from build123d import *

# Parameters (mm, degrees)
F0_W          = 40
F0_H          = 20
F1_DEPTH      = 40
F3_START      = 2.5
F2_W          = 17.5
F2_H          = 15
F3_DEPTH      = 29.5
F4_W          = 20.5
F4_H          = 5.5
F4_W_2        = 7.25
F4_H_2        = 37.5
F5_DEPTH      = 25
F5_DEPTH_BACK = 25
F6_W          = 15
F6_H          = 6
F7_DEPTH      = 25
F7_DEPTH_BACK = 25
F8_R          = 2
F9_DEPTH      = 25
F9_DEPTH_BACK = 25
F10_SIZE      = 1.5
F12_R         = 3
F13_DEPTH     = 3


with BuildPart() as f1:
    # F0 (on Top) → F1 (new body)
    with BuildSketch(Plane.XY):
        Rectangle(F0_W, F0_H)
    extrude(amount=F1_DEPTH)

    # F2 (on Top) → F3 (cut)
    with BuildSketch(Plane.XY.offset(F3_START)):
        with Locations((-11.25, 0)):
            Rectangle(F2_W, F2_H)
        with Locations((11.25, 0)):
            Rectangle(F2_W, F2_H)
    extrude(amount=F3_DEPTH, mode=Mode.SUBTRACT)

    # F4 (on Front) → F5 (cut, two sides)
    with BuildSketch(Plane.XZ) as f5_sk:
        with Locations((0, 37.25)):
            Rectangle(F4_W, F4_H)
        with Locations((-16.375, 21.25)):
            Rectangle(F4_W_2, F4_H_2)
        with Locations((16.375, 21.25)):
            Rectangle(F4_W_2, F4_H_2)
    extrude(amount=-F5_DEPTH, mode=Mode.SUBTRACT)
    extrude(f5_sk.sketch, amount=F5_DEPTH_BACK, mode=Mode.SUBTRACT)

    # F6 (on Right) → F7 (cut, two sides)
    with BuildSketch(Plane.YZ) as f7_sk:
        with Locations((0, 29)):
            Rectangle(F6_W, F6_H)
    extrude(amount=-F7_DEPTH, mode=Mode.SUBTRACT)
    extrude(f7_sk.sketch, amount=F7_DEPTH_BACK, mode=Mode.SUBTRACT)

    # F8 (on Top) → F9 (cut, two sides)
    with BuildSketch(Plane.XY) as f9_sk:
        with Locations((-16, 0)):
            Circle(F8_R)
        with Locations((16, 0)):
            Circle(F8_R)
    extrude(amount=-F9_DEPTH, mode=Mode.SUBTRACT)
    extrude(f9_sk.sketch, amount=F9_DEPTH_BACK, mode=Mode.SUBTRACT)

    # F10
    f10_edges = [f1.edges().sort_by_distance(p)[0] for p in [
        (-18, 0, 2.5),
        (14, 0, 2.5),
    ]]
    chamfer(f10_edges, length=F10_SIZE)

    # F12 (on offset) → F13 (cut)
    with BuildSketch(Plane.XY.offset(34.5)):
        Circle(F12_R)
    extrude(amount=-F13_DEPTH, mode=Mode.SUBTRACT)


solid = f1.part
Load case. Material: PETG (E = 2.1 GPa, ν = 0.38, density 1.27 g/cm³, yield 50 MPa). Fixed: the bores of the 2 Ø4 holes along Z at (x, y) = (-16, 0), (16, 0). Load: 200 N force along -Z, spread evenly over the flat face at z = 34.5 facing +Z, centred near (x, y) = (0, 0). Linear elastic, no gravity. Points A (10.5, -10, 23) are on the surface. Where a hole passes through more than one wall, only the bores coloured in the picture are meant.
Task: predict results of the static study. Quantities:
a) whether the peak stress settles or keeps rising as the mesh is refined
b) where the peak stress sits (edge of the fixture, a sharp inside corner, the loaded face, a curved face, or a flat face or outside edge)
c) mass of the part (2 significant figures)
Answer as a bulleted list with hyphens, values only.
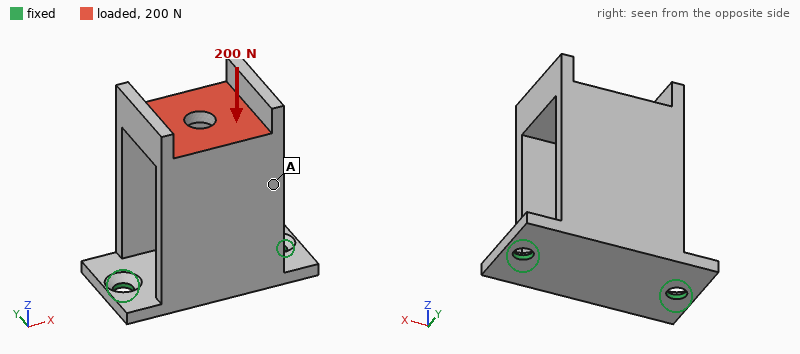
- keeps rising
- edge of the fixture
- 12 g
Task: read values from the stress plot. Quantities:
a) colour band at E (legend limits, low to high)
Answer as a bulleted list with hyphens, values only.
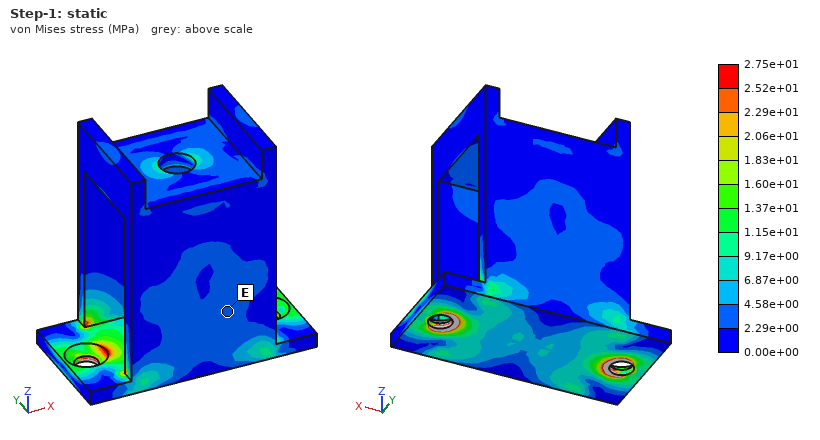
- 2.29e+00 to 4.58e+00 MPa
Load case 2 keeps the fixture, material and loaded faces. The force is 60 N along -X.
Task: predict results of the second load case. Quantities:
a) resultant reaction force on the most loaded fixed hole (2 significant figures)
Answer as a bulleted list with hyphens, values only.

- 77 N
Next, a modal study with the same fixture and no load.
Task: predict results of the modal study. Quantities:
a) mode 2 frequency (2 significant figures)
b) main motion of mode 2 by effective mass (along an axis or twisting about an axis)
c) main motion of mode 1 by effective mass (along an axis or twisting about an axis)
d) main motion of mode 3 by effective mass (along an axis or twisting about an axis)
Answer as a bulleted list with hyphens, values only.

- 820 Hz
- along X
- along Y
- along Z
